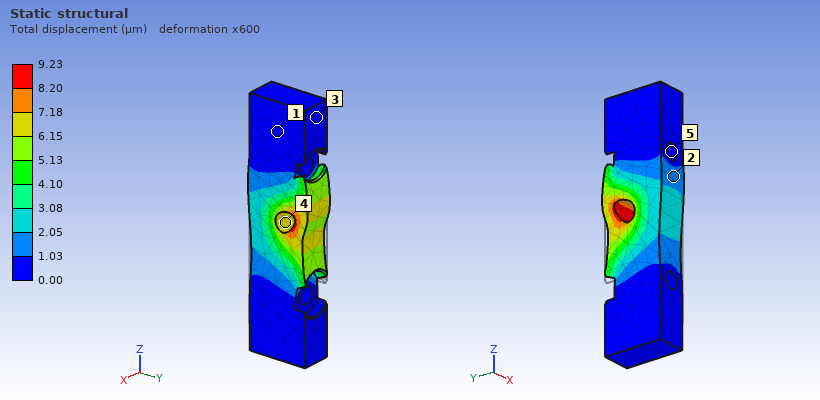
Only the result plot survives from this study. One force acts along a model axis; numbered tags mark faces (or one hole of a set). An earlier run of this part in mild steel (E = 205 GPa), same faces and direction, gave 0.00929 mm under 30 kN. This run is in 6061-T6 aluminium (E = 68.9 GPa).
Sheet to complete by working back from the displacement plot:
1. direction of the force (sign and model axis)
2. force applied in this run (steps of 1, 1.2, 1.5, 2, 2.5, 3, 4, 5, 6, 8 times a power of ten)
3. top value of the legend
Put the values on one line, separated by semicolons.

+Z; 10 kN; 9.23 µm
